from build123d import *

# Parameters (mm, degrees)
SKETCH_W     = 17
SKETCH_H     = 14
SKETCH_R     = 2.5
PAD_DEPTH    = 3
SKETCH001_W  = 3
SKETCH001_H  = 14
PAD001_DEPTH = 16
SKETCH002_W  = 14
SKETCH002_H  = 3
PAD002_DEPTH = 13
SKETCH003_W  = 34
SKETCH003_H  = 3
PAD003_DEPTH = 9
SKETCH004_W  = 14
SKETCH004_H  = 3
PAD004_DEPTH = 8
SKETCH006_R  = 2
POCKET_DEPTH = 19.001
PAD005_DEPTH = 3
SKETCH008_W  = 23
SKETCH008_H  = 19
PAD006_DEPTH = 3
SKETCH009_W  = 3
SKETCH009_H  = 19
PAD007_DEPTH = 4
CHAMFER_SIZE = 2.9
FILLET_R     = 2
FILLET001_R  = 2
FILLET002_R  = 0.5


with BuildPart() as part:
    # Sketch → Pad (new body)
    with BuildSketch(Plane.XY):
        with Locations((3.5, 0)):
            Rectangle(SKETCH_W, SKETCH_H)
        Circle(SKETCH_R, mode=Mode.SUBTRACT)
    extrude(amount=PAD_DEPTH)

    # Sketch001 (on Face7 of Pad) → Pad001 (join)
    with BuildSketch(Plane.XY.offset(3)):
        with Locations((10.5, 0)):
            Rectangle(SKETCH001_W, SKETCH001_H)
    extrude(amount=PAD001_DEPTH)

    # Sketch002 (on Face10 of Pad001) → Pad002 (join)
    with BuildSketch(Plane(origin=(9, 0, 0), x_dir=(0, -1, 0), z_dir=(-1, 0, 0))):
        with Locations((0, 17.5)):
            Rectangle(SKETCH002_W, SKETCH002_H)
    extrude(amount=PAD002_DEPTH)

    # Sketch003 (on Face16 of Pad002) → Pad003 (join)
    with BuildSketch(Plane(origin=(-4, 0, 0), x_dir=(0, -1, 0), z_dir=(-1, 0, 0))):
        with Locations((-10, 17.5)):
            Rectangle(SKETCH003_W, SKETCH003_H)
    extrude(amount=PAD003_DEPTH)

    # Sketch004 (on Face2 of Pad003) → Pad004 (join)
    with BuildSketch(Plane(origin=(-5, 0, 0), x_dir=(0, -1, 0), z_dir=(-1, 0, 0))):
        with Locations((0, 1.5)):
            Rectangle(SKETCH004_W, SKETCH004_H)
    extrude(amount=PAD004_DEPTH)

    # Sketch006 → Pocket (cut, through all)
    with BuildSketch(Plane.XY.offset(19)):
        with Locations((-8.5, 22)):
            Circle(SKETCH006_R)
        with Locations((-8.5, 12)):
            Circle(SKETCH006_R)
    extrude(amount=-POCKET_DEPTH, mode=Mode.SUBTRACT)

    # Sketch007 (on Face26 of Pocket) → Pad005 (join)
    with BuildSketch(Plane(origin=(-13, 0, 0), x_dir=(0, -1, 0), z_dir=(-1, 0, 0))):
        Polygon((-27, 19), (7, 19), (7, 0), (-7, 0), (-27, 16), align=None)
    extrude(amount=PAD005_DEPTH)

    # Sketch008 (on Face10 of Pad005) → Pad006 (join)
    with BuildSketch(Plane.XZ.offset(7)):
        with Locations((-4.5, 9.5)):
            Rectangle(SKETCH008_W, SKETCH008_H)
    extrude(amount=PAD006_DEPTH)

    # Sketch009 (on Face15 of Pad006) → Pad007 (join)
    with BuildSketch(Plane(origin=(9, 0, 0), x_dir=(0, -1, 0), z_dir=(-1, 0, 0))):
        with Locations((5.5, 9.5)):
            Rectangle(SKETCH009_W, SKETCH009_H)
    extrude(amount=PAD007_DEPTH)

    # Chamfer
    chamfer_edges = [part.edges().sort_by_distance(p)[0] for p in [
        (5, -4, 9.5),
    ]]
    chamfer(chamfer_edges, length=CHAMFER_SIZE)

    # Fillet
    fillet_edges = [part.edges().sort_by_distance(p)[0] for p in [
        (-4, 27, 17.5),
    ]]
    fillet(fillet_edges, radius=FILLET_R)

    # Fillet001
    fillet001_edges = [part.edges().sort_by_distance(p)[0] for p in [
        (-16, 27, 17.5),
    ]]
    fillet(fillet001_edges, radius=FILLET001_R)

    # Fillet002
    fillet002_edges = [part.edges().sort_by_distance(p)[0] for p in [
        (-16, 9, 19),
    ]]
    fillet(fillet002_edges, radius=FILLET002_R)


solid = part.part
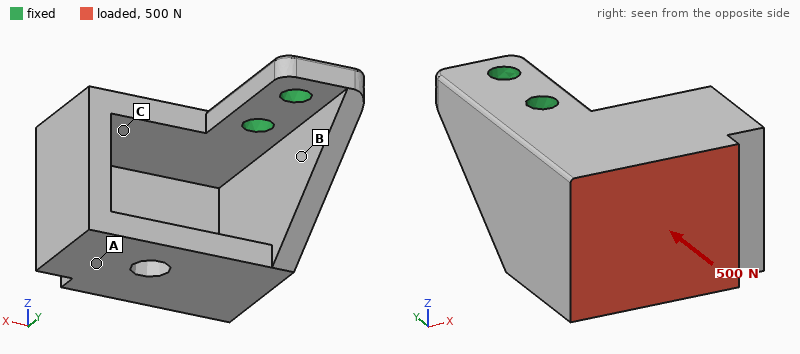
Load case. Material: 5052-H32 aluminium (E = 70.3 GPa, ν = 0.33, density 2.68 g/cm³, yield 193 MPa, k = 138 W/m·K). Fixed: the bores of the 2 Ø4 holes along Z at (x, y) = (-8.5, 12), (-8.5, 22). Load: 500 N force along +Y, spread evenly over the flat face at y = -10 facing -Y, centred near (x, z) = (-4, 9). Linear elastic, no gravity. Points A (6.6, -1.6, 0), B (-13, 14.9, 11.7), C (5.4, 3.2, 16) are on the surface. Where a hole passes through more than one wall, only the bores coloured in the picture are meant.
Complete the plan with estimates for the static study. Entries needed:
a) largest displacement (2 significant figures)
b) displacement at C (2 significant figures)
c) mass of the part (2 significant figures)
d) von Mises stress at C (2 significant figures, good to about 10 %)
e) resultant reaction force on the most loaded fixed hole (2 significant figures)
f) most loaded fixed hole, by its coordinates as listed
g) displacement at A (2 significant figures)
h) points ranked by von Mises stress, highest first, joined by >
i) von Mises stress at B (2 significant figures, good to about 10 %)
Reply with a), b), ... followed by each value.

a) 98 µm
b) 31 µm
c) 16 g
d) 15 MPa
e) 540 N
f) (-8.5, 12)
g) 83 µm
h) B > C > A
i) 28 MPa
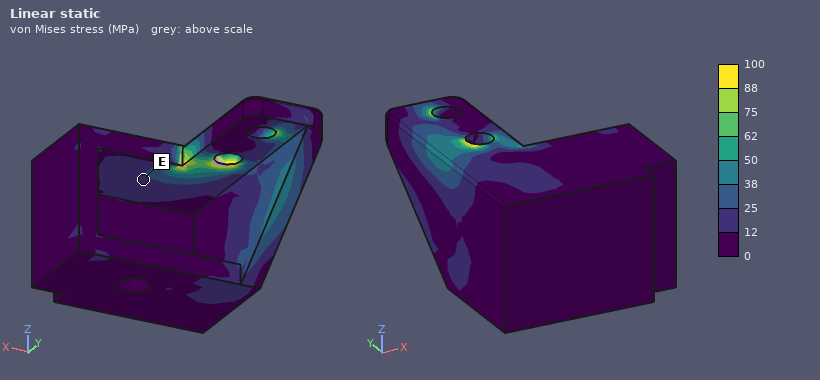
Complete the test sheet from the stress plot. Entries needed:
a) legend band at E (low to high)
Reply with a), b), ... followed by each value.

a) 12 to 25 MPa
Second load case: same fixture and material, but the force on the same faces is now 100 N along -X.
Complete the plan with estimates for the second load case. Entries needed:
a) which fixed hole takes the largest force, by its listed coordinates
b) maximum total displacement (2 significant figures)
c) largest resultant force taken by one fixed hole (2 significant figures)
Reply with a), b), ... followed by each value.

a) (-8.5, 12)
b) 52 µm
c) 220 N
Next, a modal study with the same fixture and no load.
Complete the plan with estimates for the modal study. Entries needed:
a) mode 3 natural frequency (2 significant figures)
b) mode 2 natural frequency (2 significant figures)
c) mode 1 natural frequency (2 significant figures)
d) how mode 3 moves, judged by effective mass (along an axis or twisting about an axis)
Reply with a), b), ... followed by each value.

a) 5900 Hz
b) 3100 Hz
c) 2000 Hz
d) along Z
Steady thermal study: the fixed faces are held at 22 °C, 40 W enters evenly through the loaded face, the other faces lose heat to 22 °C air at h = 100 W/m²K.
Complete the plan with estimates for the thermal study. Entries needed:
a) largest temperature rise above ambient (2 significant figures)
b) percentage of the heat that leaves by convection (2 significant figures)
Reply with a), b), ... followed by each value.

a) 57 K
b) 36 %
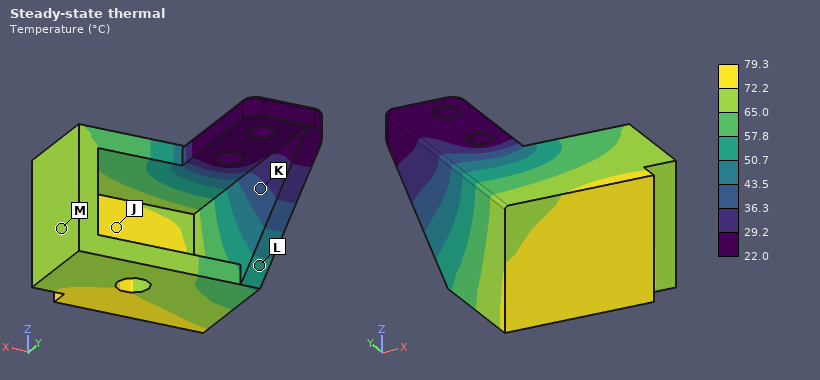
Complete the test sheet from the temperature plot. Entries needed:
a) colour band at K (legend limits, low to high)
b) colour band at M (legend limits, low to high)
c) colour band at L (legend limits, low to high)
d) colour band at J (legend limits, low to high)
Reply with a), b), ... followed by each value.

a) 36.3 to 43.5 °C
b) 65.0 to 72.2 °C
c) 50.7 to 57.8 °C
d) 72.2 to 79.3 °C
